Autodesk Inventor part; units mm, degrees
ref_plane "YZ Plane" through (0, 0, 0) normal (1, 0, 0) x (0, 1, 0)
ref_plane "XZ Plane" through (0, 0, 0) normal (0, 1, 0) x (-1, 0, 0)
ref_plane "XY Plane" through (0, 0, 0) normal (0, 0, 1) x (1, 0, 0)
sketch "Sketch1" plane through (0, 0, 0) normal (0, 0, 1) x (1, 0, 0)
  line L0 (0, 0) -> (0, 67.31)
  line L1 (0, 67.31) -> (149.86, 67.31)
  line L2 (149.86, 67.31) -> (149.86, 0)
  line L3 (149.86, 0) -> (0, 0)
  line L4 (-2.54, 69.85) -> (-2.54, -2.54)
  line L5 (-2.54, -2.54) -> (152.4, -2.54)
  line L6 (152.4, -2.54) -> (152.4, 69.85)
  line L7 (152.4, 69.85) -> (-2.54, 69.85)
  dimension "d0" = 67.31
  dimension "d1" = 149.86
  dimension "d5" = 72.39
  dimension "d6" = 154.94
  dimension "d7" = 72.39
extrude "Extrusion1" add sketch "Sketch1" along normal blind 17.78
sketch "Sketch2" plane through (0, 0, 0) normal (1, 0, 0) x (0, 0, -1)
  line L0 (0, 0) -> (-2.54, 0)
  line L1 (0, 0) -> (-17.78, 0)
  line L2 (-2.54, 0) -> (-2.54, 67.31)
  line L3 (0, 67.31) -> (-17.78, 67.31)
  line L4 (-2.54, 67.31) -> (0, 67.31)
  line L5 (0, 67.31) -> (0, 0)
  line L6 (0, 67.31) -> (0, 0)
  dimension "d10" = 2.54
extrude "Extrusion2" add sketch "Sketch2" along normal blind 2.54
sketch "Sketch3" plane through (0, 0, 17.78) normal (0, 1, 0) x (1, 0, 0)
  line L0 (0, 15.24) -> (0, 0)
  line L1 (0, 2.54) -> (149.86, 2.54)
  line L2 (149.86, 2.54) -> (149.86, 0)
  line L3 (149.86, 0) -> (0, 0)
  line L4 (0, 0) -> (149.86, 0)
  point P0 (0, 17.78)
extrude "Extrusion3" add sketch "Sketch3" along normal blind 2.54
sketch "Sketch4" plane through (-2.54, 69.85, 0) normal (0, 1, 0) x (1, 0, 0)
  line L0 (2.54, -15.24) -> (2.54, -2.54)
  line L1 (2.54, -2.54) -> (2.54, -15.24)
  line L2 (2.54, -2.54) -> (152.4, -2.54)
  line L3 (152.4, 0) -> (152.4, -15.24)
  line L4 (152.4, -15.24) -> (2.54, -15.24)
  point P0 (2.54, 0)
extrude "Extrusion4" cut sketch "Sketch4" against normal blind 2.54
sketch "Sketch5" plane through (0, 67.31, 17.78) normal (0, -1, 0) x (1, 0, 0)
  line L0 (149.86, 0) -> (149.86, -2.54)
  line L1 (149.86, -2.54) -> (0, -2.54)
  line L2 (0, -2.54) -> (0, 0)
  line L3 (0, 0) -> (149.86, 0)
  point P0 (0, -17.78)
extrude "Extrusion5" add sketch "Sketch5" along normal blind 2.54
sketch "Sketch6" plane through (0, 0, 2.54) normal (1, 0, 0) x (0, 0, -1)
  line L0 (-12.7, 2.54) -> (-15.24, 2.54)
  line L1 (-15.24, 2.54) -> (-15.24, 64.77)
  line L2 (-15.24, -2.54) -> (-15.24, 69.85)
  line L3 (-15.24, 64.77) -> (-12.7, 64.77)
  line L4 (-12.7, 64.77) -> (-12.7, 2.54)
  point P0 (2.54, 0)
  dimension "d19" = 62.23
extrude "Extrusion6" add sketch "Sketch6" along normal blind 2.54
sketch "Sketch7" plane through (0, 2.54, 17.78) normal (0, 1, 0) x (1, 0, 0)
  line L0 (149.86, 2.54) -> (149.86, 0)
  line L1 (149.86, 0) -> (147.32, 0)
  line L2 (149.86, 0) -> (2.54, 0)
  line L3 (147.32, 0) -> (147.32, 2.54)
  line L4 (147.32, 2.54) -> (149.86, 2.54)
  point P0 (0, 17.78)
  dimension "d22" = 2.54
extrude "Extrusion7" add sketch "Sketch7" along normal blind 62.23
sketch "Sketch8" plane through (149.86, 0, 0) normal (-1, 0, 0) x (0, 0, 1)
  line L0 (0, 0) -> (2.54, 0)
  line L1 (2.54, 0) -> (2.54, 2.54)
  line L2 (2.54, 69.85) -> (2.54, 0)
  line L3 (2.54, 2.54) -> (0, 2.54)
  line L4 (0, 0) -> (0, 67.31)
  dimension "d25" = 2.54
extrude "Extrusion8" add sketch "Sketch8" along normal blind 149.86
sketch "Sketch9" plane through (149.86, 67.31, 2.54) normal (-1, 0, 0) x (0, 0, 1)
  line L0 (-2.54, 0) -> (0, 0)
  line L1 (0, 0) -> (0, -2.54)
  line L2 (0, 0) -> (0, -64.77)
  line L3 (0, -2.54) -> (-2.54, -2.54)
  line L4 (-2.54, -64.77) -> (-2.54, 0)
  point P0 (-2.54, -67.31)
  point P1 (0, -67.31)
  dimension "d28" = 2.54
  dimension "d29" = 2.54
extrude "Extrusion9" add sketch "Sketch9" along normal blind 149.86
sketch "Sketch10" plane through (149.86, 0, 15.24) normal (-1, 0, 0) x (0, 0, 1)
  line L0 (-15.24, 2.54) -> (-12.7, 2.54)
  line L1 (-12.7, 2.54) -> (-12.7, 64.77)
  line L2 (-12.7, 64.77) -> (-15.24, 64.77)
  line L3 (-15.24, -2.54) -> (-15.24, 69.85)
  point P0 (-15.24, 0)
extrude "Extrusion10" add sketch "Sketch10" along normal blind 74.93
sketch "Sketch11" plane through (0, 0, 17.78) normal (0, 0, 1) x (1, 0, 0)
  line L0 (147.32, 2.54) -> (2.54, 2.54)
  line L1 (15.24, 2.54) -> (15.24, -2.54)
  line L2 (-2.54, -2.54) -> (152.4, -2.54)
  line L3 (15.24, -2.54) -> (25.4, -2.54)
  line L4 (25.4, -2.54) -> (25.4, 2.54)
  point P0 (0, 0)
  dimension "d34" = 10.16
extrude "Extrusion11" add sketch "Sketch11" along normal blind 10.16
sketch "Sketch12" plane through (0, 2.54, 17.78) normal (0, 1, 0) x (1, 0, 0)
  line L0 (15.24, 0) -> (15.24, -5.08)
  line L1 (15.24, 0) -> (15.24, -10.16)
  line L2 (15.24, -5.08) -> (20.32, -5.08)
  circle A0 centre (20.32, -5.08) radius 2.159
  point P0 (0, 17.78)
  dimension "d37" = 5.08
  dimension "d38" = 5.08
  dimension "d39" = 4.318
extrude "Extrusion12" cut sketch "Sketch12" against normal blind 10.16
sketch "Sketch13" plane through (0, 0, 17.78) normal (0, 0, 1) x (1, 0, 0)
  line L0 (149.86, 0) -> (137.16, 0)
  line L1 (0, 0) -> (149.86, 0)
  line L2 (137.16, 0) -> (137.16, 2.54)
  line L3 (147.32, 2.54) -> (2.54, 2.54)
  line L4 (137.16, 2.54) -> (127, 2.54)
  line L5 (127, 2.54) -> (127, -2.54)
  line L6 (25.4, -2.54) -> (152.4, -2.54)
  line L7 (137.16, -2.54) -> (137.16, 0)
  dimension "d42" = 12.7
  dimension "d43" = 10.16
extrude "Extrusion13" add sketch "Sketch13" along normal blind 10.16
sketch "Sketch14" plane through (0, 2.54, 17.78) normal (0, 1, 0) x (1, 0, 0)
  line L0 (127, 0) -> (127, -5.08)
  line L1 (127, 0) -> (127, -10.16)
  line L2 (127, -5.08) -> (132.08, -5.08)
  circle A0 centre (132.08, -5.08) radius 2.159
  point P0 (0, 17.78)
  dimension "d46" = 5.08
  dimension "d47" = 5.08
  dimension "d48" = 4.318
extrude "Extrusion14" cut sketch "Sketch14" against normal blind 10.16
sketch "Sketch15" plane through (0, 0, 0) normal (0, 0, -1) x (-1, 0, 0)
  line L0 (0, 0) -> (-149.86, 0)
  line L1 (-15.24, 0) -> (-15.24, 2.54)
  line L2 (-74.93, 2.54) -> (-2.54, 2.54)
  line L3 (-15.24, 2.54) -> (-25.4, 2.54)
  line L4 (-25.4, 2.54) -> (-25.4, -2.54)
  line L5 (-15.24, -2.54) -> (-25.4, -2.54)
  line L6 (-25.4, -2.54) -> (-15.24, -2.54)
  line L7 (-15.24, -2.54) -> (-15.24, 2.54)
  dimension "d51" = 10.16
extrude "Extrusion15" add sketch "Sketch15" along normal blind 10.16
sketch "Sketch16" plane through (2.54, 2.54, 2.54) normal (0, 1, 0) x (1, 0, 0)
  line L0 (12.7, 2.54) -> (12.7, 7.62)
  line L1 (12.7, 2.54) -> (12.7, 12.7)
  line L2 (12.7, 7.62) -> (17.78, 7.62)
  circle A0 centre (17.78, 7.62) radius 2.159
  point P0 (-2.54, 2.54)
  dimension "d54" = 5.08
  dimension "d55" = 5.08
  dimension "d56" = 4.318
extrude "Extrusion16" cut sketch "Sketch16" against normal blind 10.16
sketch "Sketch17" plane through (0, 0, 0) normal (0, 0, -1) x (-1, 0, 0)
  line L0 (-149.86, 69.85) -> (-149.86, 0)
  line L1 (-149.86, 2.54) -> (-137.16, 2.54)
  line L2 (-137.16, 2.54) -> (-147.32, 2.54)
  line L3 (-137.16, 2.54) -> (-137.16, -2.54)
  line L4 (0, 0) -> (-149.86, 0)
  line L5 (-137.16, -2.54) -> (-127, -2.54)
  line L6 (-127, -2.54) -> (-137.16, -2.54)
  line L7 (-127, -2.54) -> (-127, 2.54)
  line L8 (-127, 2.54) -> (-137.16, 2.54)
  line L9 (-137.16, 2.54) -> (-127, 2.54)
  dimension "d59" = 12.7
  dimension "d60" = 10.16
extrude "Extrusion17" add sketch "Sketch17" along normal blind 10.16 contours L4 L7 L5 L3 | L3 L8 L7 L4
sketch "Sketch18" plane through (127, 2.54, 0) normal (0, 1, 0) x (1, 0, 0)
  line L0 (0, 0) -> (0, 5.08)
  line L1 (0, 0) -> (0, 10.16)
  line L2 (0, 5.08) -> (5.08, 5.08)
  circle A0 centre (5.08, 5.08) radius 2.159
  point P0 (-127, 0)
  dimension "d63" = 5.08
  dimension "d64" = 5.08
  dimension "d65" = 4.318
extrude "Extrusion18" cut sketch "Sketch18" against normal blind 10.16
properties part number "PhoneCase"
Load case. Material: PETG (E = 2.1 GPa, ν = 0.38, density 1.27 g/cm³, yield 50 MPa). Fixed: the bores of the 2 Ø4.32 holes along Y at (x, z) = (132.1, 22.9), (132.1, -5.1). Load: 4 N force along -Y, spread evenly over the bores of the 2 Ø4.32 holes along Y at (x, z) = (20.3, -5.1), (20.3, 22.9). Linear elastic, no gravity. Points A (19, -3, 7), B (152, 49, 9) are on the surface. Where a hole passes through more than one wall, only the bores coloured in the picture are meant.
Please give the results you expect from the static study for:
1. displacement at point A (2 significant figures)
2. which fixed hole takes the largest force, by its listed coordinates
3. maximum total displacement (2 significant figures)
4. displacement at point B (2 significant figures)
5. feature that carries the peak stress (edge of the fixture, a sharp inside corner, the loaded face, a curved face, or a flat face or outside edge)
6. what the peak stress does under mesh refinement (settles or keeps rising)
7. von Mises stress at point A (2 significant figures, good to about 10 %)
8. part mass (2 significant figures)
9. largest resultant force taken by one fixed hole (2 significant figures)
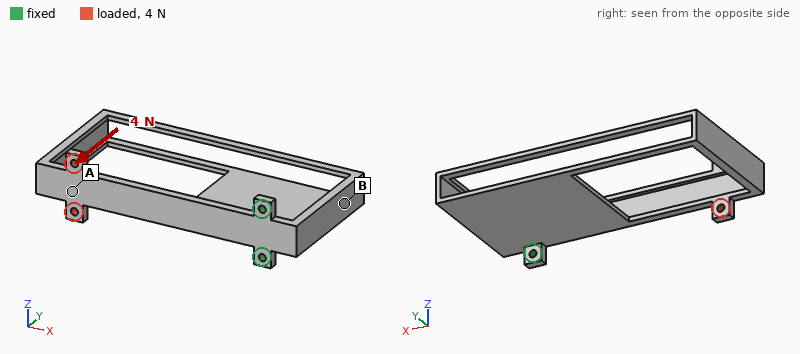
1.4 mm
(132.1, -5.1)
1.9 mm
0.37 mm
edge of the fixture
keeps rising
0.99 MPa
43 g
3.5 N
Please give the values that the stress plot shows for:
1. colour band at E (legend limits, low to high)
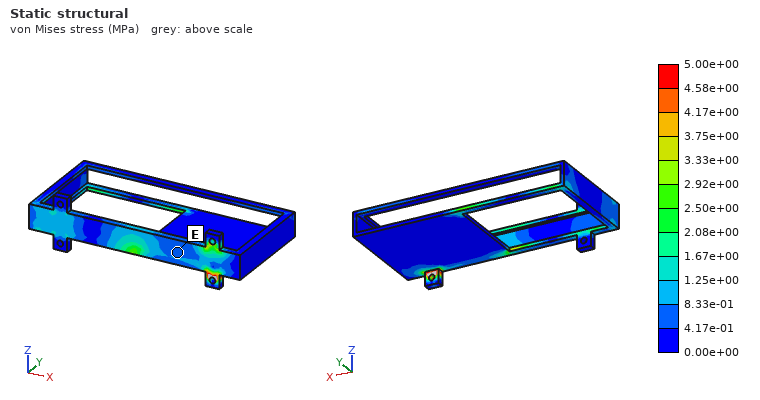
4.17e-01 to 8.33e-01 MPa
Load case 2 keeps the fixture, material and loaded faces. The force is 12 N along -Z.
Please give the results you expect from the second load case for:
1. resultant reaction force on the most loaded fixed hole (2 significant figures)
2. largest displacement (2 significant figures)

59 N
1.9 mm
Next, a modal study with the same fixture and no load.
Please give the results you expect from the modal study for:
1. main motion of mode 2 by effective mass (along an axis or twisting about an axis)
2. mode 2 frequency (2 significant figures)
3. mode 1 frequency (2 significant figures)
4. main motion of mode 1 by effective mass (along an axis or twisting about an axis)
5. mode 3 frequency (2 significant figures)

along Y
67 Hz
52 Hz
along Z
150 Hz
